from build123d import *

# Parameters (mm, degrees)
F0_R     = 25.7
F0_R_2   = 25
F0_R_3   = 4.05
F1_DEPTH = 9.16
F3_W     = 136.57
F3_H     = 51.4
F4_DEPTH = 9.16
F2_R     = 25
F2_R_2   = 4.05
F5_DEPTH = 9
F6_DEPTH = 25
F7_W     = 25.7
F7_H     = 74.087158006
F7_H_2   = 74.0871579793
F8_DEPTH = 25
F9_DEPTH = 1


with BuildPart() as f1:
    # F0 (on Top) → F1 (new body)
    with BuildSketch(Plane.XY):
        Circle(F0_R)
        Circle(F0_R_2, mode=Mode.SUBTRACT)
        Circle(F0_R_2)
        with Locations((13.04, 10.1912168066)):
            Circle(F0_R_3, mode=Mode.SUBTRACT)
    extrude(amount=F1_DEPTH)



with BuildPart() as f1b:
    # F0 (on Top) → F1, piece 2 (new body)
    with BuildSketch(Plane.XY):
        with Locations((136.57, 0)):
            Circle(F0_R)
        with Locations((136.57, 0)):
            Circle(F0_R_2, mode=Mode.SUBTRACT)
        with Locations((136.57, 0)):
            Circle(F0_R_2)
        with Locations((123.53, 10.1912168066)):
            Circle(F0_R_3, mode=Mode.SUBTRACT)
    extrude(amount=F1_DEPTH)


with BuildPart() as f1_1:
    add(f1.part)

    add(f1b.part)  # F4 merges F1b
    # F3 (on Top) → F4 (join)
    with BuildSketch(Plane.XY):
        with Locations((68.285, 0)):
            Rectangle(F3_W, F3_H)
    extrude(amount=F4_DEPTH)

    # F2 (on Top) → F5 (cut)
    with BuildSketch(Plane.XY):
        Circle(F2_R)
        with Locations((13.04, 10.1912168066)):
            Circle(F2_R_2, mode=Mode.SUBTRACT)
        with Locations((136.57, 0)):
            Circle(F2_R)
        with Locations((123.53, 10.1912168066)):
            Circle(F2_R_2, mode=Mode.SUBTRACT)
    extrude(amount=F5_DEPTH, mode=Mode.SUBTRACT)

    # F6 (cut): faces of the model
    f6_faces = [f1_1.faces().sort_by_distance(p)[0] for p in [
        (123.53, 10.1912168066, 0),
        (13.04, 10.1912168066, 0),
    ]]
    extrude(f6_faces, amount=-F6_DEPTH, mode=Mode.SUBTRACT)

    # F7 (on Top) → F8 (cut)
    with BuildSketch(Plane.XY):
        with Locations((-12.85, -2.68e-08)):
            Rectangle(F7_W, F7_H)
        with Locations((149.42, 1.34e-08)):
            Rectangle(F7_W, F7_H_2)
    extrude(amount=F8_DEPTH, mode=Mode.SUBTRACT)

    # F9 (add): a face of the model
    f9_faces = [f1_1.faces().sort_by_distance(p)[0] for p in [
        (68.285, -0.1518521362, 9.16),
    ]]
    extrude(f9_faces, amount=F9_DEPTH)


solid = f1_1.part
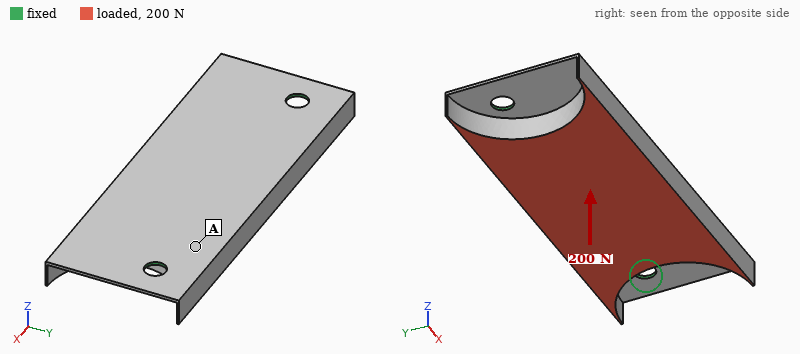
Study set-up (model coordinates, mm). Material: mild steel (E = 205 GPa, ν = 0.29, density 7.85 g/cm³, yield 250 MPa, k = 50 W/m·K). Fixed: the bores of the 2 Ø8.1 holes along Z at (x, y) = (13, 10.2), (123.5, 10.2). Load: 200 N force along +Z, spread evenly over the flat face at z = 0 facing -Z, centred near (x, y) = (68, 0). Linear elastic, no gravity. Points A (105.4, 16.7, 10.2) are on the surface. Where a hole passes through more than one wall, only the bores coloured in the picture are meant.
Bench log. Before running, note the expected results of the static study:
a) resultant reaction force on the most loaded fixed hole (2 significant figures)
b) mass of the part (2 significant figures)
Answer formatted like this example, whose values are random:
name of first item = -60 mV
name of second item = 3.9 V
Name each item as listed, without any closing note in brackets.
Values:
resultant reaction force on the most loaded fixed hole = 160 N
mass of the part = 420 g
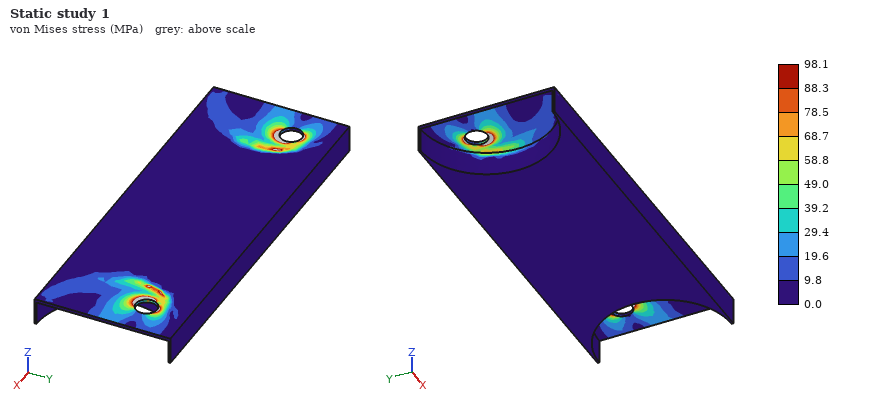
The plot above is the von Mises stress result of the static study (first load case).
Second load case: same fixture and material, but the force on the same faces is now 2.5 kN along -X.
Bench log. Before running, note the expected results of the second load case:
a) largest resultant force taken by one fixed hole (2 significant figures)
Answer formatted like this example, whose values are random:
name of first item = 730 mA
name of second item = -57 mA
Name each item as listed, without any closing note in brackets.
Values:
largest resultant force taken by one fixed hole = 1.3 kN
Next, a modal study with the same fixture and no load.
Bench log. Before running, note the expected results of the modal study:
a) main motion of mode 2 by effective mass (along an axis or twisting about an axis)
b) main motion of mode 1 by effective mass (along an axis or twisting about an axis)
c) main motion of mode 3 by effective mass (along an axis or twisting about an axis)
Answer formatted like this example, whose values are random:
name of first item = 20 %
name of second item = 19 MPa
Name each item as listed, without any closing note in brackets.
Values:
main motion of mode 2 by effective mass = along Z
main motion of mode 1 by effective mass = along Z
main motion of mode 3 by effective mass = twisting about Y
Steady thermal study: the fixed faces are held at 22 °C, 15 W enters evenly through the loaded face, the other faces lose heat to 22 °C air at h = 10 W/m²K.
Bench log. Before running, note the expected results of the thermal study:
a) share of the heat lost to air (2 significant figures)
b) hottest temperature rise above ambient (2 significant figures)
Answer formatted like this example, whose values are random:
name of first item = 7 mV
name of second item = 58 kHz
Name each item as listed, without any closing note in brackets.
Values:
share of the heat lost to air = 22 %
hottest temperature rise above ambient = 33 K
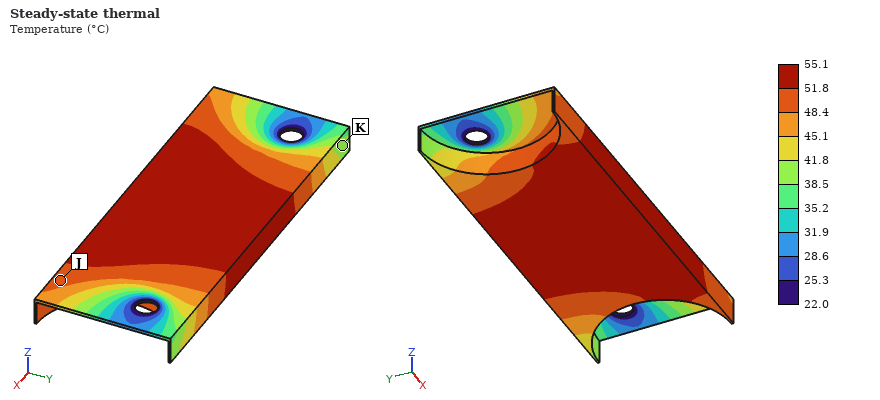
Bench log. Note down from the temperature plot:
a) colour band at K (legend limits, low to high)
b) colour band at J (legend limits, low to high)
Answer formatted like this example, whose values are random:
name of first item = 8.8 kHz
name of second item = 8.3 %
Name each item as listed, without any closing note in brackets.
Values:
colour band at K = 38.5 to 41.8 °C
colour band at J = 48.4 to 51.8 °C
